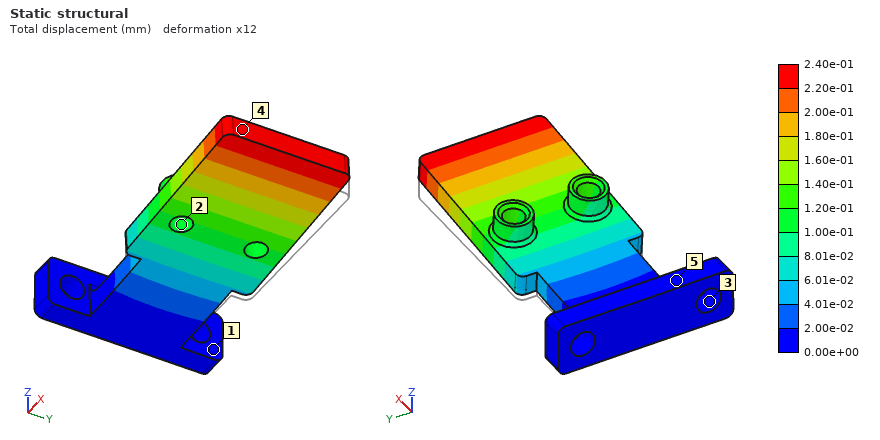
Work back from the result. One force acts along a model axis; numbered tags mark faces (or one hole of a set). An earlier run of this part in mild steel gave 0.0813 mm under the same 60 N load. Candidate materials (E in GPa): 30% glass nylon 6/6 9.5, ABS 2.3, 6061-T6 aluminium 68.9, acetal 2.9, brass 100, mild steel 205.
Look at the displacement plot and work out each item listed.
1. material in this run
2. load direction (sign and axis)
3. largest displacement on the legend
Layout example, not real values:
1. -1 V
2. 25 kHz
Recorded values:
1. 6061-T6 aluminium
2. +Z
3. 2.40e-01 mm
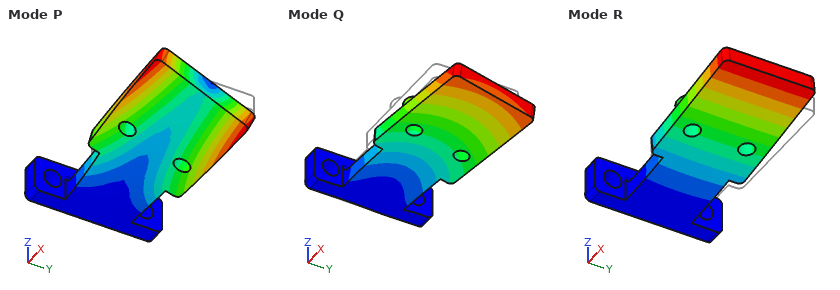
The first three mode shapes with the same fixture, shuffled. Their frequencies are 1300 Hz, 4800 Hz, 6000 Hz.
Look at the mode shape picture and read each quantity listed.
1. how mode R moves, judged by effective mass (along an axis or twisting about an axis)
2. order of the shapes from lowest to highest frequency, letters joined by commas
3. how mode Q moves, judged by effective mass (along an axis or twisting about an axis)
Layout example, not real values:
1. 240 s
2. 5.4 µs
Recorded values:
1. along Z
2. R, Q, P
3. along Y
